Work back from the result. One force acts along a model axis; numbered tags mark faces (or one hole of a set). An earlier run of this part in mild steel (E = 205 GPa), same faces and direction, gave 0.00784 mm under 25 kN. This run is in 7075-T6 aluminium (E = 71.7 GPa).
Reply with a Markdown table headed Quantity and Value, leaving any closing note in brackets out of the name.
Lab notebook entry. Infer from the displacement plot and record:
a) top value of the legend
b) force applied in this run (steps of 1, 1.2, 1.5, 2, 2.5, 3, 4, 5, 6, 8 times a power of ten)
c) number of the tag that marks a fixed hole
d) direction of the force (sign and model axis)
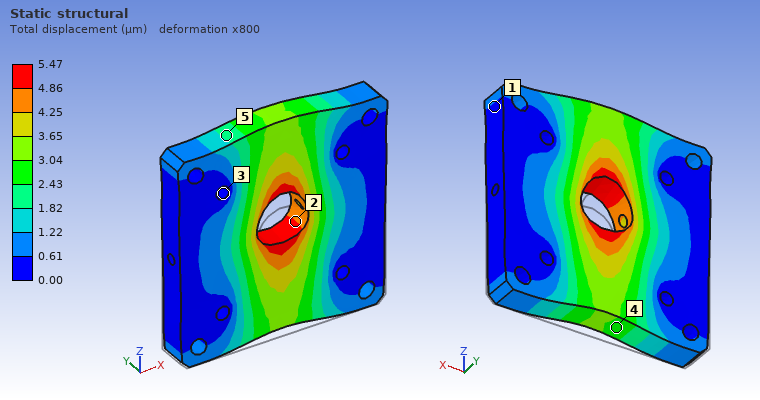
| Quantity | Value |
|---|---|
| top value of the legend | 5.47 µm |
| force applied in this run | 6 kN |
| number of the tag that marks a fixed hole | 3 |
| direction of the force | +Z |
